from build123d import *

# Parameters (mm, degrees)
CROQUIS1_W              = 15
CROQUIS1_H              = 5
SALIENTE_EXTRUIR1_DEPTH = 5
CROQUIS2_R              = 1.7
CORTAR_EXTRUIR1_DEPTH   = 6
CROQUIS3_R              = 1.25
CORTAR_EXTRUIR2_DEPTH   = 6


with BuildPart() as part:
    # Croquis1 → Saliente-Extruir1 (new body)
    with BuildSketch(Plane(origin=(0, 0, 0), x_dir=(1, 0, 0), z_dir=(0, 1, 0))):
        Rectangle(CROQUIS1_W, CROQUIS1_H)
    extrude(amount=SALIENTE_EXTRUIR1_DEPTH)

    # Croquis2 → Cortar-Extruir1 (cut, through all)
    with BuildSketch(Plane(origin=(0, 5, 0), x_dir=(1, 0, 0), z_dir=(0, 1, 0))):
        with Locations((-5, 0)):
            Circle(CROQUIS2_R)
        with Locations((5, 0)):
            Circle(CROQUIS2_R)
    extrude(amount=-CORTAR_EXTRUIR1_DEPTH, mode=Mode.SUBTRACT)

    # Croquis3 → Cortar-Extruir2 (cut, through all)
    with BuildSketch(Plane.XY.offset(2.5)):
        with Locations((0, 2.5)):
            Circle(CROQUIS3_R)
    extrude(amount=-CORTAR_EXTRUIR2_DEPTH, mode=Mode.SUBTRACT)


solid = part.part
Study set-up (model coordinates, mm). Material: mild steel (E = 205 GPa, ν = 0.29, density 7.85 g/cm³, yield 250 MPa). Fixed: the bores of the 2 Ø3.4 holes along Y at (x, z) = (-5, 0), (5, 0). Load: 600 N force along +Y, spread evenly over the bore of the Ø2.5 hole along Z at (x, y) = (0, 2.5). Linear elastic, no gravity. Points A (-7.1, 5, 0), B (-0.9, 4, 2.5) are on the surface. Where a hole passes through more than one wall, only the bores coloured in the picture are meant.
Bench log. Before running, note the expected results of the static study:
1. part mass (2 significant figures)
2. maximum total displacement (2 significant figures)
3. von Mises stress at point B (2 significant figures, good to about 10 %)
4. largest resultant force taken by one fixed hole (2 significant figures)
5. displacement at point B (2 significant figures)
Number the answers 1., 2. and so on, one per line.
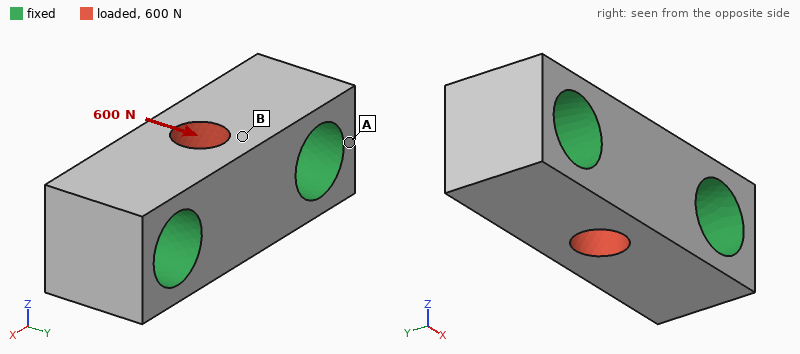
1. 2.0 g
2. 0.76 µm
3. 22 MPa
4. 300 N
5. 0.59 µm
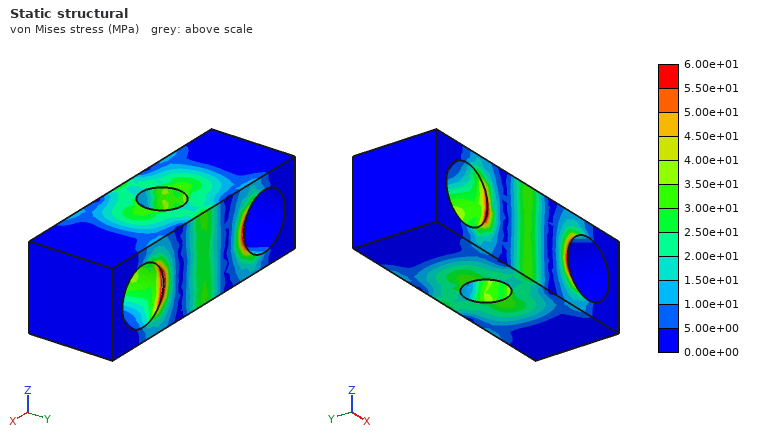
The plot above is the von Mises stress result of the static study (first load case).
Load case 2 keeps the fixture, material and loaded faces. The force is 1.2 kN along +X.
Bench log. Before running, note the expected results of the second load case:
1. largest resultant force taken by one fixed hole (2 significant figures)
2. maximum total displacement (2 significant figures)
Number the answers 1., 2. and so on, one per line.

1. 600 N
2. 0.48 µm
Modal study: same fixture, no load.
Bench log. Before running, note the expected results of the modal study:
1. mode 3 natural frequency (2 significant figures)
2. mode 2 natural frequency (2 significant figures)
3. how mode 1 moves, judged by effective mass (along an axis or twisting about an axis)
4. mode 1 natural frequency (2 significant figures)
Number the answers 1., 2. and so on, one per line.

1. 210 kHz
2. 210 kHz
3. along Z
4. 190 kHz
